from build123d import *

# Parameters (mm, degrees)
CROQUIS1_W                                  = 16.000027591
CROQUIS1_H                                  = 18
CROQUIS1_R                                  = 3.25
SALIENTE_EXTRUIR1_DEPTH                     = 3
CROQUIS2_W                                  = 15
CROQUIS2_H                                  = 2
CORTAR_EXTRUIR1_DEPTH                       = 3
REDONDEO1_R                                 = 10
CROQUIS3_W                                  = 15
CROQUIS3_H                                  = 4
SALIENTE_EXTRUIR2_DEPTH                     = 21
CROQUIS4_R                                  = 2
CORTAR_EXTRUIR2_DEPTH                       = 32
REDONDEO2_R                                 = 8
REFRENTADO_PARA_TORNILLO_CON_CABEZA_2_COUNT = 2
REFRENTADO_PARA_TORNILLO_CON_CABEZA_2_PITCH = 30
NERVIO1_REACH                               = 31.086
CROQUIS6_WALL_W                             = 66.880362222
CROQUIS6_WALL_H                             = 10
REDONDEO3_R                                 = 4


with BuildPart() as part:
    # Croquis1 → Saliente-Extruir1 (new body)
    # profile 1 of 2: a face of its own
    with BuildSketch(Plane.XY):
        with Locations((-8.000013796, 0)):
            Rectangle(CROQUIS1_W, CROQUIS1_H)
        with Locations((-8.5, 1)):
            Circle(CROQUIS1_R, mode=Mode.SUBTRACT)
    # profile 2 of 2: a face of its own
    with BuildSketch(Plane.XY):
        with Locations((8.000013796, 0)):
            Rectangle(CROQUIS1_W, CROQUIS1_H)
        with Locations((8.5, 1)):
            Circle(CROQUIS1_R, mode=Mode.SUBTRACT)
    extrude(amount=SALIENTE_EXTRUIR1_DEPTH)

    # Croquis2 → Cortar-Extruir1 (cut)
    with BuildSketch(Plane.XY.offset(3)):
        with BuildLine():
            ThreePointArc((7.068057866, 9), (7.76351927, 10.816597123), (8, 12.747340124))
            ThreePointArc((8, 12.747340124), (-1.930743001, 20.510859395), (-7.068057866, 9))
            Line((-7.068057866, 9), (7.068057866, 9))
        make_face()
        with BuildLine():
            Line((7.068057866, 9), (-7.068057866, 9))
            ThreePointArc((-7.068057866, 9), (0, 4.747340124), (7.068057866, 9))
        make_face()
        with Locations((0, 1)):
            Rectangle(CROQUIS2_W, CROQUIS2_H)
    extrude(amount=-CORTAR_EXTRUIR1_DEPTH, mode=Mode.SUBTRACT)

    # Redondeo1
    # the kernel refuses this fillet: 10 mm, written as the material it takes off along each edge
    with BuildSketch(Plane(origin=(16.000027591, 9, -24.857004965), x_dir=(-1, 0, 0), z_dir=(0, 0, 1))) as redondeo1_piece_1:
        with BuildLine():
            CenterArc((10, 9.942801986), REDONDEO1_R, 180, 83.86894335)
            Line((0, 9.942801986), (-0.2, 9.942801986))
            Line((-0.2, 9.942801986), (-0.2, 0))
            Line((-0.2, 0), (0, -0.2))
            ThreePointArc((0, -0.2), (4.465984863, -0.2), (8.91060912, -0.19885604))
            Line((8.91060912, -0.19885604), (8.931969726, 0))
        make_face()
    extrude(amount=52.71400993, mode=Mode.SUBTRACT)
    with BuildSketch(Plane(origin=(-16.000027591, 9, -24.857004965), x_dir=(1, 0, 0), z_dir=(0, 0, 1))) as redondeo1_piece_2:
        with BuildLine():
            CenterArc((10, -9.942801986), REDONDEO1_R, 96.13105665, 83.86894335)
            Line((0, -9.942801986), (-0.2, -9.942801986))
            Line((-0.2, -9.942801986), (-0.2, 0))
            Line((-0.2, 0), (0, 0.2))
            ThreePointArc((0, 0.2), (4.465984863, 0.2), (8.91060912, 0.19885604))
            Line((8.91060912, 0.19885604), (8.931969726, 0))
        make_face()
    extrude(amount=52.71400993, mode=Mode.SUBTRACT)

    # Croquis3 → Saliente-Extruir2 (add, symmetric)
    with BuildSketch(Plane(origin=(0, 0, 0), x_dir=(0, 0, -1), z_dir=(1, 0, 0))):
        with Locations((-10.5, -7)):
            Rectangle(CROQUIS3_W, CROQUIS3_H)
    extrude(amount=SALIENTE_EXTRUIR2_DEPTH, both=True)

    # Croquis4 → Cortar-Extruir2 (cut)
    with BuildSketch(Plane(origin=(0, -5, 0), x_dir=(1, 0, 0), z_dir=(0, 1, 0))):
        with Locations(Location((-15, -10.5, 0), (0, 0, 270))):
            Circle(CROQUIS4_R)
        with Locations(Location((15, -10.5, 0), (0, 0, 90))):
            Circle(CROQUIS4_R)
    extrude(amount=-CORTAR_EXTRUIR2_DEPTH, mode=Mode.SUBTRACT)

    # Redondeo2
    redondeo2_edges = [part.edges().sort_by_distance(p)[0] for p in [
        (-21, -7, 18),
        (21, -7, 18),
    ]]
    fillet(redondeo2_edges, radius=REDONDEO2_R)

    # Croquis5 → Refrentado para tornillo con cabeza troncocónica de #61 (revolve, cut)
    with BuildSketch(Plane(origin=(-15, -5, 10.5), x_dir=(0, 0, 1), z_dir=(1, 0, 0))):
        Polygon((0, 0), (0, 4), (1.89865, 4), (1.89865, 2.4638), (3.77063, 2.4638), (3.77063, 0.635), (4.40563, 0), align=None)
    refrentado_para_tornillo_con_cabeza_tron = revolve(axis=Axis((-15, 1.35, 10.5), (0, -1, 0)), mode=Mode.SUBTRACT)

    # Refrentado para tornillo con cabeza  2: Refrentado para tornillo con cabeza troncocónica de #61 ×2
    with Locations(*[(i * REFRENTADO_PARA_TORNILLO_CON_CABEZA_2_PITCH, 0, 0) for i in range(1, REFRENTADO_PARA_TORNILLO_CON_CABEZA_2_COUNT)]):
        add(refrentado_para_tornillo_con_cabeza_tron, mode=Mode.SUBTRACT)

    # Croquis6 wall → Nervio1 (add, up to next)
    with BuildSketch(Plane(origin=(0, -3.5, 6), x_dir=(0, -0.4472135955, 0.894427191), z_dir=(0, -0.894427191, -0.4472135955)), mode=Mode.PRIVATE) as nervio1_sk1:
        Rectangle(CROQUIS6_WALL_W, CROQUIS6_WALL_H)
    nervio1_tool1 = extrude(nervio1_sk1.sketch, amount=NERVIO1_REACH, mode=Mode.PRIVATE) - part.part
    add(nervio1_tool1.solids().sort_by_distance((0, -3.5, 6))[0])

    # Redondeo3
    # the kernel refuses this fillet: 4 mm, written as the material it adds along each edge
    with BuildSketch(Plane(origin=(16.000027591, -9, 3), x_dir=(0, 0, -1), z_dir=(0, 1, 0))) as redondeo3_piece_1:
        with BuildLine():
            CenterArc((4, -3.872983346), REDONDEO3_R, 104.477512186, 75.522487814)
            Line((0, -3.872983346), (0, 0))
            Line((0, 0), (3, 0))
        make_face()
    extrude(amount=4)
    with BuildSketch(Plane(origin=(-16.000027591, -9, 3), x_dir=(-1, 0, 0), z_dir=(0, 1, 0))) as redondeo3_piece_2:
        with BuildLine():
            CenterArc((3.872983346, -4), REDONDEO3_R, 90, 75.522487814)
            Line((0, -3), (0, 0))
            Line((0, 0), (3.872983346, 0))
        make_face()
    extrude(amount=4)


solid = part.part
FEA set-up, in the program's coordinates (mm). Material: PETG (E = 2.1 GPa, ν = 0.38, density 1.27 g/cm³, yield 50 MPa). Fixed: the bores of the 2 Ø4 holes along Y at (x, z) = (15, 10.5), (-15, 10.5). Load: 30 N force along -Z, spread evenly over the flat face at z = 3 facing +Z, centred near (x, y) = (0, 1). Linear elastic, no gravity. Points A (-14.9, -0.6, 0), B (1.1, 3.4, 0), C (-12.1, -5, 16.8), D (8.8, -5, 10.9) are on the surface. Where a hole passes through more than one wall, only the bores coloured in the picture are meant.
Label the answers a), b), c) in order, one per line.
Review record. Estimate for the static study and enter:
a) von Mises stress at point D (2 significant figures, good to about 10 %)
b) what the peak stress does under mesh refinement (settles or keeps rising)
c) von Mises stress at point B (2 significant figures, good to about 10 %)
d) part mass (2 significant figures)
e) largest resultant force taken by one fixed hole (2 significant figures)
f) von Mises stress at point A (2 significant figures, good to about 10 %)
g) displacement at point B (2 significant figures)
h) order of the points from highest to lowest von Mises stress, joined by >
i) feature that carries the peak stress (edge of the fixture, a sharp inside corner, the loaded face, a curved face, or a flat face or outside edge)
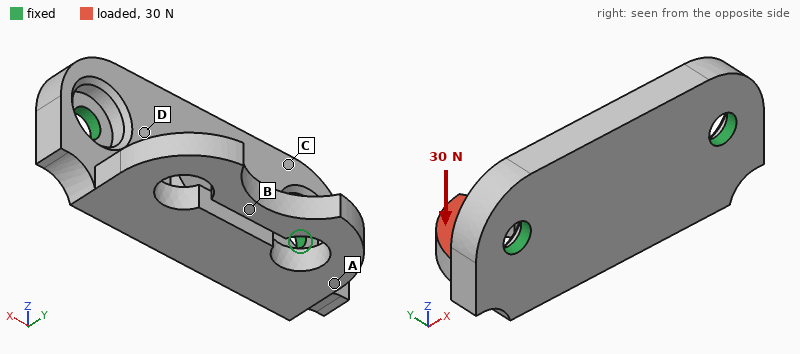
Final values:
a) 3.0 MPa
b) keeps rising
c) 4.5 MPa
d) 4.4 g
e) 15 N
f) 6.5 MPa
g) 0.39 mm
h) A > B > D > C
i) edge of the fixture
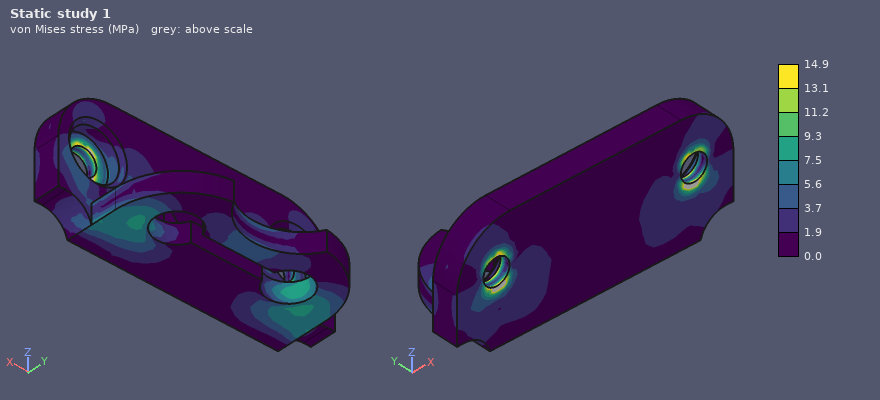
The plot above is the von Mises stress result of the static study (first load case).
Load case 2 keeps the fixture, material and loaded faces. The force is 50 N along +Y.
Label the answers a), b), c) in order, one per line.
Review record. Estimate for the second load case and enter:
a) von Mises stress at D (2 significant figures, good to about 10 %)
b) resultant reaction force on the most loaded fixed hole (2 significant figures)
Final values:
a) 2.7 MPa
b) 27 N
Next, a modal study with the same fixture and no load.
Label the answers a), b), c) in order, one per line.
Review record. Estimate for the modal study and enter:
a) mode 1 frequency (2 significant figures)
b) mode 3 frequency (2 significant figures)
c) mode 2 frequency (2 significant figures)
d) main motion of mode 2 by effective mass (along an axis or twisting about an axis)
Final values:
a) 1400 Hz
b) 2900 Hz
c) 2700 Hz
d) along Y
